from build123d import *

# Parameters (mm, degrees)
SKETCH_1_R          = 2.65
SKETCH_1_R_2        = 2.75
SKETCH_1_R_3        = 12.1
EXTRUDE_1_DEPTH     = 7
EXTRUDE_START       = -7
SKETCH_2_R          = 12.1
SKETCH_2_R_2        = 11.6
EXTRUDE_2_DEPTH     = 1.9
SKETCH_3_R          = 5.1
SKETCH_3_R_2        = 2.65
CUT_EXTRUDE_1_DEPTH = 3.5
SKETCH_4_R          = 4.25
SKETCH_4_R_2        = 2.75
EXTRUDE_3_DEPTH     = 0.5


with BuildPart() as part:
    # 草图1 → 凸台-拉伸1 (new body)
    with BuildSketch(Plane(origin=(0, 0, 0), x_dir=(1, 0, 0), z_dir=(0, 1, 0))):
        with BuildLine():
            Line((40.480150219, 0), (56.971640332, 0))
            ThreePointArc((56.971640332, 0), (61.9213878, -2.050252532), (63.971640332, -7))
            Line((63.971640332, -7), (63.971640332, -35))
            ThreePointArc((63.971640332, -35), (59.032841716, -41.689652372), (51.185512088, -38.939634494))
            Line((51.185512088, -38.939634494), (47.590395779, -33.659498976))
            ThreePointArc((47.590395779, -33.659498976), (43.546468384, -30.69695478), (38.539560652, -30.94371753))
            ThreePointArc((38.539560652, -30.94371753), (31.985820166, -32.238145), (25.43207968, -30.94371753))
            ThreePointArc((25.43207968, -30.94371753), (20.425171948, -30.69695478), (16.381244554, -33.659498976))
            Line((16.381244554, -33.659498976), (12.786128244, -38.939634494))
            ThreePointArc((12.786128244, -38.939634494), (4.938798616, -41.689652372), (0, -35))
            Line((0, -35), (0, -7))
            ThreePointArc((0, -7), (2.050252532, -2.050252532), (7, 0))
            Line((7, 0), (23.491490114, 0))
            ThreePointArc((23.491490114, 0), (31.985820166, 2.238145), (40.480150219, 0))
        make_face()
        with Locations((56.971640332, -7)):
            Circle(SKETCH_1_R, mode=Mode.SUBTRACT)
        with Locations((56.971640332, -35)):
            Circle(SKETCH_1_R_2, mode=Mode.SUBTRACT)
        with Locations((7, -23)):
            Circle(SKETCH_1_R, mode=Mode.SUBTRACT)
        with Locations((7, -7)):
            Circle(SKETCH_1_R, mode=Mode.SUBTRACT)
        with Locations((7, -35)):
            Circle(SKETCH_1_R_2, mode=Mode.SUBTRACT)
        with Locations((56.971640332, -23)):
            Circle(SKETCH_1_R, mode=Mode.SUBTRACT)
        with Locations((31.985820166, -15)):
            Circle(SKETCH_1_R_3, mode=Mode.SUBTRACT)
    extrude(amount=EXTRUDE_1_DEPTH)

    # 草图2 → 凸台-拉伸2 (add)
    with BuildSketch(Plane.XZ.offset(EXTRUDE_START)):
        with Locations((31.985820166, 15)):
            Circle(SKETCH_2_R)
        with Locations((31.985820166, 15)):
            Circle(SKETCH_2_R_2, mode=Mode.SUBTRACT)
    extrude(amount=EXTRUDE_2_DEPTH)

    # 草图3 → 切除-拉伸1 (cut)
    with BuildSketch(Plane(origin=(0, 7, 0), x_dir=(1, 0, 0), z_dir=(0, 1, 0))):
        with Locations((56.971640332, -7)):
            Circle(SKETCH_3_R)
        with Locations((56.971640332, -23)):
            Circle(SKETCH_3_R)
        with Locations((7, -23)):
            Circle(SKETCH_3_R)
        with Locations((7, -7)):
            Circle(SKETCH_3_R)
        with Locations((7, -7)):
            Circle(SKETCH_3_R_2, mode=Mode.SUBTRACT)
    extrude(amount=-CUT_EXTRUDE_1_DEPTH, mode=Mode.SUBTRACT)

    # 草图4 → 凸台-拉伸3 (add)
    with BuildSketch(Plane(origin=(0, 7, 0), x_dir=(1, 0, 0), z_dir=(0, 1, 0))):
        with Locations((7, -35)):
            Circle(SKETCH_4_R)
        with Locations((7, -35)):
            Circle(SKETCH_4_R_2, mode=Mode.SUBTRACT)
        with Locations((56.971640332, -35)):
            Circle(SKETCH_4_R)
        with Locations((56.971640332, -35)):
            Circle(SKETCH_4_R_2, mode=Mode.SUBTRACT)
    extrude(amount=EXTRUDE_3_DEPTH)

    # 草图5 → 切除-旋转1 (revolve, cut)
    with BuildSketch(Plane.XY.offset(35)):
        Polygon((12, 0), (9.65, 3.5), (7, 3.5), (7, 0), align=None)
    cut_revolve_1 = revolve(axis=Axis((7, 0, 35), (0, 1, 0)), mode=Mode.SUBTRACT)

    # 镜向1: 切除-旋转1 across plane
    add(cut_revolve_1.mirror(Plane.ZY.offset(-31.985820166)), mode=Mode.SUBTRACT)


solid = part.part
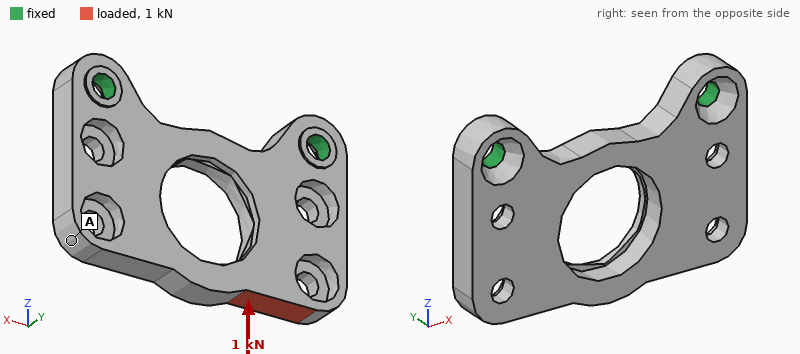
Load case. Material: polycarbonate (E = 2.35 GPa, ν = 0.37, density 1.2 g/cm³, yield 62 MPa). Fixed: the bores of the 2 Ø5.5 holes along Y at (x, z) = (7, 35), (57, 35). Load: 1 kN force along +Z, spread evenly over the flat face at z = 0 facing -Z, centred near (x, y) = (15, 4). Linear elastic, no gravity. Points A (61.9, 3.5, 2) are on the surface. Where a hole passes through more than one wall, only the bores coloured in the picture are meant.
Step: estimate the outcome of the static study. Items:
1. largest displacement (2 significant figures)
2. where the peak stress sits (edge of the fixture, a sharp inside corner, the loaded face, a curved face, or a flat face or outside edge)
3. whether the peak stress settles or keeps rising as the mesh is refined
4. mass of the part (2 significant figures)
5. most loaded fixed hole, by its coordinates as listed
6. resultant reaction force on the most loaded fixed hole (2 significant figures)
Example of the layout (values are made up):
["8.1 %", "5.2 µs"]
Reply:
["0.28 mm", "edge of the fixture", "keeps rising", "13 g", "(7, 35)", "890 N"]
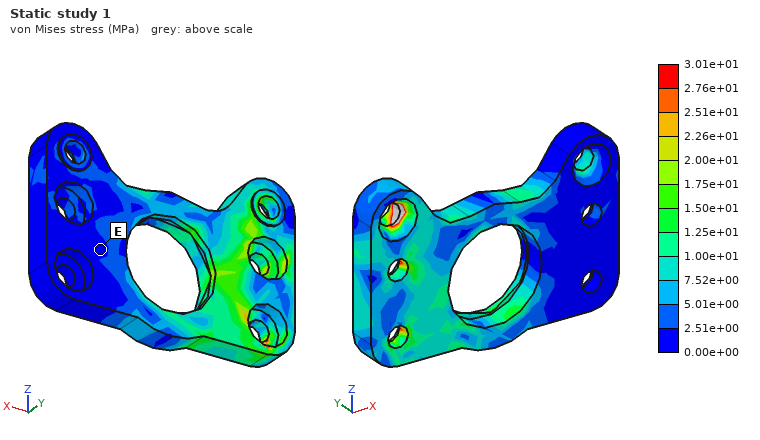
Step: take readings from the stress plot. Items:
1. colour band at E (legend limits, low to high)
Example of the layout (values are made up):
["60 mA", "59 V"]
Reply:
["0.00e+00 to 2.51e+00 MPa"]
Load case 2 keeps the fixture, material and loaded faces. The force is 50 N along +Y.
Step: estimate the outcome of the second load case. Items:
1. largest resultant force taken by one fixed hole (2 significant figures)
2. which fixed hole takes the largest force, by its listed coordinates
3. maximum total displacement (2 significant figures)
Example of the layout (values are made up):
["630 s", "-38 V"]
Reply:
["41 N", "(7, 35)", "0.67 mm"]
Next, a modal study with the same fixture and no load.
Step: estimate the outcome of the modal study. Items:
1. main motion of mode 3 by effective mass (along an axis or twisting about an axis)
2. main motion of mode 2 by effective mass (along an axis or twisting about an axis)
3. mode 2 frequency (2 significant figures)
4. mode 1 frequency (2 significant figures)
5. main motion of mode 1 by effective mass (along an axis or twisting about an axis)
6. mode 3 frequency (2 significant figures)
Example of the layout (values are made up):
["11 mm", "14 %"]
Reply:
["along X", "twisting about Z", "1600 Hz", "830 Hz", "along Y", "2500 Hz"]
